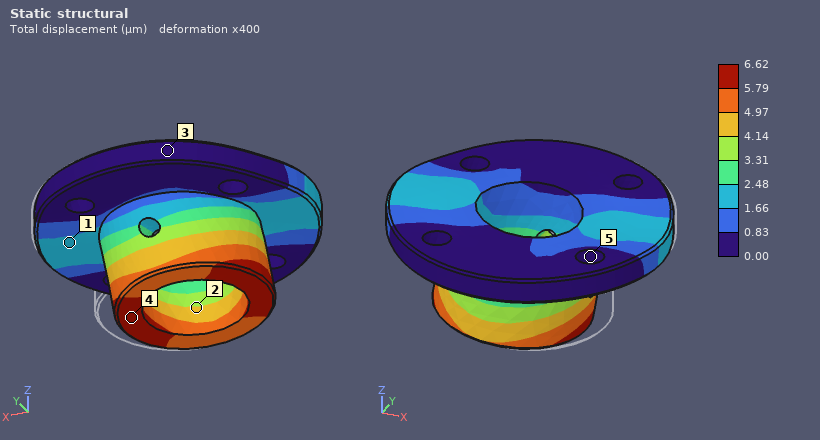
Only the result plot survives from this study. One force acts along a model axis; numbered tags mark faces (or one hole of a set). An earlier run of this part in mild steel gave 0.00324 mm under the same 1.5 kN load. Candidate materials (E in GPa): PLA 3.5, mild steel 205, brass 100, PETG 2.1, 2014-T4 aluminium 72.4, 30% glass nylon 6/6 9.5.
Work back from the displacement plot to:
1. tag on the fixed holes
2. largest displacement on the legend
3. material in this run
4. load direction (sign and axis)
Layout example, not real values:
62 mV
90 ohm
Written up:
5
6.62 µm
brass
-X
